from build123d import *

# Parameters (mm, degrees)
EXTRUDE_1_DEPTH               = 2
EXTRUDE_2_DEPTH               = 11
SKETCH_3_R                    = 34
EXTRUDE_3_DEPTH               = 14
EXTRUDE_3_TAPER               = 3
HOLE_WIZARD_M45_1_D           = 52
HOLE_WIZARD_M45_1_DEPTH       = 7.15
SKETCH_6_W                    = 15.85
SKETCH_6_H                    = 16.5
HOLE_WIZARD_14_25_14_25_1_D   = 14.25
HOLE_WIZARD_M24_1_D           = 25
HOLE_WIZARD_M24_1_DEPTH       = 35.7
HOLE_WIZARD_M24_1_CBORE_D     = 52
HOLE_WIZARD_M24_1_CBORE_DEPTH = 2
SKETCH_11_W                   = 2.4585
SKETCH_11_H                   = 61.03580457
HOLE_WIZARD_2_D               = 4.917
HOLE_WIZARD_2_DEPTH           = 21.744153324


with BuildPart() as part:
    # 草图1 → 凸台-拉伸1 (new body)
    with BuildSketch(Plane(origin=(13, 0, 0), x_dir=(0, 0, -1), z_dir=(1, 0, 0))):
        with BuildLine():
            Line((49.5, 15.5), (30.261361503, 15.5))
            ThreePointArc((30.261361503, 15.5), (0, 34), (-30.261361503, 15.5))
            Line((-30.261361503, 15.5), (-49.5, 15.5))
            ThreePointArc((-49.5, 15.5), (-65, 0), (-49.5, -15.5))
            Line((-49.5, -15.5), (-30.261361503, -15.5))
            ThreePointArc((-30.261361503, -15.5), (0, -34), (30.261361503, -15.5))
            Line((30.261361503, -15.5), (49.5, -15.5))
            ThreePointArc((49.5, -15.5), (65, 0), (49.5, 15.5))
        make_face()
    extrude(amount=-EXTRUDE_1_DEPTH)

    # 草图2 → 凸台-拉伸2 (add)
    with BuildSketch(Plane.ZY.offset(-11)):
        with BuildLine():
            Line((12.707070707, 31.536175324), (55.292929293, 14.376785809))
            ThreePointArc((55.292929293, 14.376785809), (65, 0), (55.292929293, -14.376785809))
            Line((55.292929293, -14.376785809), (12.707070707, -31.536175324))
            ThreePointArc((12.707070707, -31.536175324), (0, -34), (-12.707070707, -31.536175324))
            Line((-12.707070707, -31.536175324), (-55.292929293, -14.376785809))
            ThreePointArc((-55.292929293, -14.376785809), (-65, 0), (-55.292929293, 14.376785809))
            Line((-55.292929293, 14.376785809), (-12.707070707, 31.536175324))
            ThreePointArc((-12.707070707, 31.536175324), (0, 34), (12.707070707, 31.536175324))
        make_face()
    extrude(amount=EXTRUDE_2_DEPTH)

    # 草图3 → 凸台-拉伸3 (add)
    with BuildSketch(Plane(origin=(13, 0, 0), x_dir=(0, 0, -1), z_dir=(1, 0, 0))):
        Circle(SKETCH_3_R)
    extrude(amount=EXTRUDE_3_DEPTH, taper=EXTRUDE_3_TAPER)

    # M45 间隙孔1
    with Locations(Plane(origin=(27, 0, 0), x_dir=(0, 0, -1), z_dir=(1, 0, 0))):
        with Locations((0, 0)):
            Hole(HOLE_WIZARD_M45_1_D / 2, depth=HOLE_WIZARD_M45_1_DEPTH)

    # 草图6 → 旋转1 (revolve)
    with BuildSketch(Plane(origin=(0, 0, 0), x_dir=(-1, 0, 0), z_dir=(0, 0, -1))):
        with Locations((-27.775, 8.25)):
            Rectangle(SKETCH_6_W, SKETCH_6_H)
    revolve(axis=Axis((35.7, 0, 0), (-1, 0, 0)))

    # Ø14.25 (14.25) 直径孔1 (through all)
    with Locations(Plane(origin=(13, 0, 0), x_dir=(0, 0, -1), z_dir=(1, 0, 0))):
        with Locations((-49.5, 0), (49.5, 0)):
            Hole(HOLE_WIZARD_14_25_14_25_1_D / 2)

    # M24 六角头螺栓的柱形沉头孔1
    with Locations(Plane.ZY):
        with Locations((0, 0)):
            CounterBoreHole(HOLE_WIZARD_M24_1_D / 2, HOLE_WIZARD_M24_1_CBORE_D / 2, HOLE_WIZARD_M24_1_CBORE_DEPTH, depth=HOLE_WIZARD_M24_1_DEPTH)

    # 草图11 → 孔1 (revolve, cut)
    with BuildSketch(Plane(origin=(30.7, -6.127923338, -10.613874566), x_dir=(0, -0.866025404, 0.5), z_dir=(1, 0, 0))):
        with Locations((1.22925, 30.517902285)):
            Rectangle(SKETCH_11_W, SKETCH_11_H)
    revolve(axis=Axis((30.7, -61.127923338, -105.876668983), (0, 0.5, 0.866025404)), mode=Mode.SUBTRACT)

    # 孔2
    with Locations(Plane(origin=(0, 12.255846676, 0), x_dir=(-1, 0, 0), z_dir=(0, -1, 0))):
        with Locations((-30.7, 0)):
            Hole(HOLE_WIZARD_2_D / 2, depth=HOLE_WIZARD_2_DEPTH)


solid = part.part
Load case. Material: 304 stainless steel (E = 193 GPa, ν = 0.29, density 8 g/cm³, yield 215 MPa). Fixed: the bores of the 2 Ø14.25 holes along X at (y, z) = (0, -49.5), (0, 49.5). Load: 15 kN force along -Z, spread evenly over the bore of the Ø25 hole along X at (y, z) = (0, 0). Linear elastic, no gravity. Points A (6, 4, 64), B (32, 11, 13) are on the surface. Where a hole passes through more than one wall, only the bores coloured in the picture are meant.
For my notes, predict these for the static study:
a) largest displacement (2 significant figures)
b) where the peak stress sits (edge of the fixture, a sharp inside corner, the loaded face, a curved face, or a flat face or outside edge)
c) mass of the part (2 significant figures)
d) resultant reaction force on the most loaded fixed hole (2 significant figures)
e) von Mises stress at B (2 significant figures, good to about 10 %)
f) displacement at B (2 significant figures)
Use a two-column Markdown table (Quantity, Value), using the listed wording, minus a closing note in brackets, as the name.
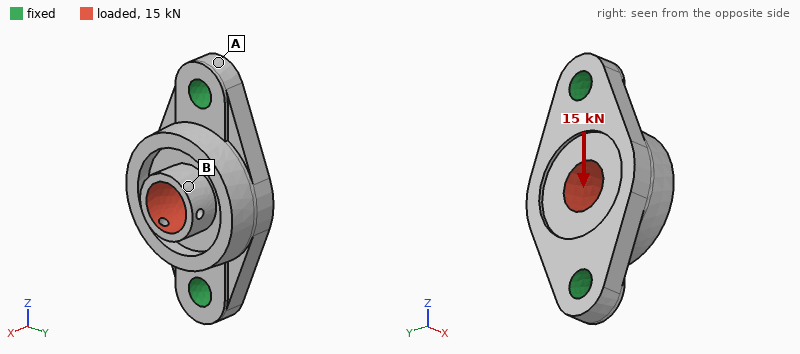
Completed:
| Quantity | Value |
|---|---|
| largest displacement | 13 µm |
| where the peak stress sits | the loaded face |
| mass of the part | 800 g |
| resultant reaction force on the most loaded fixed hole | 7.9 kN |
| von Mises stress at B | 18 MPa |
| displacement at B | 10 µm |
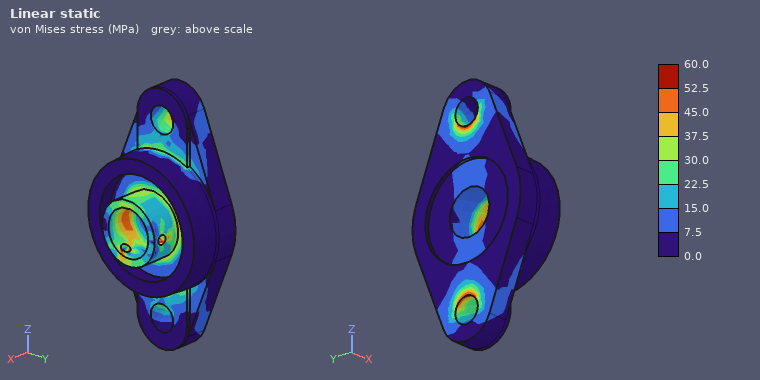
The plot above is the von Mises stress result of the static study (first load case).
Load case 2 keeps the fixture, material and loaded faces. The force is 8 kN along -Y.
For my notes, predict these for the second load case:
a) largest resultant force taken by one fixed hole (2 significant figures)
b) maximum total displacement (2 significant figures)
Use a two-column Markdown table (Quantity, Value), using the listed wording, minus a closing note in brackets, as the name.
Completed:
| Quantity | Value |
|---|---|
| largest resultant force taken by one fixed hole | 4.0 kN |
| maximum total displacement | 23 µm |
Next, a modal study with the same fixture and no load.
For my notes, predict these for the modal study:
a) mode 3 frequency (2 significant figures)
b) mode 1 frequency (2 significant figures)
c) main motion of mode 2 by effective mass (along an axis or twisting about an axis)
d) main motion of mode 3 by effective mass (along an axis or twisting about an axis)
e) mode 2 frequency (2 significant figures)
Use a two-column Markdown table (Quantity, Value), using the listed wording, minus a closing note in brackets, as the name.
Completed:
| Quantity | Value |
|---|---|
| mode 3 frequency | 11 kHz |
| mode 1 frequency | 4400 Hz |
| main motion of mode 2 by effective mass | along X |
| main motion of mode 3 by effective mass | along Y |
| mode 2 frequency | 5900 Hz |
